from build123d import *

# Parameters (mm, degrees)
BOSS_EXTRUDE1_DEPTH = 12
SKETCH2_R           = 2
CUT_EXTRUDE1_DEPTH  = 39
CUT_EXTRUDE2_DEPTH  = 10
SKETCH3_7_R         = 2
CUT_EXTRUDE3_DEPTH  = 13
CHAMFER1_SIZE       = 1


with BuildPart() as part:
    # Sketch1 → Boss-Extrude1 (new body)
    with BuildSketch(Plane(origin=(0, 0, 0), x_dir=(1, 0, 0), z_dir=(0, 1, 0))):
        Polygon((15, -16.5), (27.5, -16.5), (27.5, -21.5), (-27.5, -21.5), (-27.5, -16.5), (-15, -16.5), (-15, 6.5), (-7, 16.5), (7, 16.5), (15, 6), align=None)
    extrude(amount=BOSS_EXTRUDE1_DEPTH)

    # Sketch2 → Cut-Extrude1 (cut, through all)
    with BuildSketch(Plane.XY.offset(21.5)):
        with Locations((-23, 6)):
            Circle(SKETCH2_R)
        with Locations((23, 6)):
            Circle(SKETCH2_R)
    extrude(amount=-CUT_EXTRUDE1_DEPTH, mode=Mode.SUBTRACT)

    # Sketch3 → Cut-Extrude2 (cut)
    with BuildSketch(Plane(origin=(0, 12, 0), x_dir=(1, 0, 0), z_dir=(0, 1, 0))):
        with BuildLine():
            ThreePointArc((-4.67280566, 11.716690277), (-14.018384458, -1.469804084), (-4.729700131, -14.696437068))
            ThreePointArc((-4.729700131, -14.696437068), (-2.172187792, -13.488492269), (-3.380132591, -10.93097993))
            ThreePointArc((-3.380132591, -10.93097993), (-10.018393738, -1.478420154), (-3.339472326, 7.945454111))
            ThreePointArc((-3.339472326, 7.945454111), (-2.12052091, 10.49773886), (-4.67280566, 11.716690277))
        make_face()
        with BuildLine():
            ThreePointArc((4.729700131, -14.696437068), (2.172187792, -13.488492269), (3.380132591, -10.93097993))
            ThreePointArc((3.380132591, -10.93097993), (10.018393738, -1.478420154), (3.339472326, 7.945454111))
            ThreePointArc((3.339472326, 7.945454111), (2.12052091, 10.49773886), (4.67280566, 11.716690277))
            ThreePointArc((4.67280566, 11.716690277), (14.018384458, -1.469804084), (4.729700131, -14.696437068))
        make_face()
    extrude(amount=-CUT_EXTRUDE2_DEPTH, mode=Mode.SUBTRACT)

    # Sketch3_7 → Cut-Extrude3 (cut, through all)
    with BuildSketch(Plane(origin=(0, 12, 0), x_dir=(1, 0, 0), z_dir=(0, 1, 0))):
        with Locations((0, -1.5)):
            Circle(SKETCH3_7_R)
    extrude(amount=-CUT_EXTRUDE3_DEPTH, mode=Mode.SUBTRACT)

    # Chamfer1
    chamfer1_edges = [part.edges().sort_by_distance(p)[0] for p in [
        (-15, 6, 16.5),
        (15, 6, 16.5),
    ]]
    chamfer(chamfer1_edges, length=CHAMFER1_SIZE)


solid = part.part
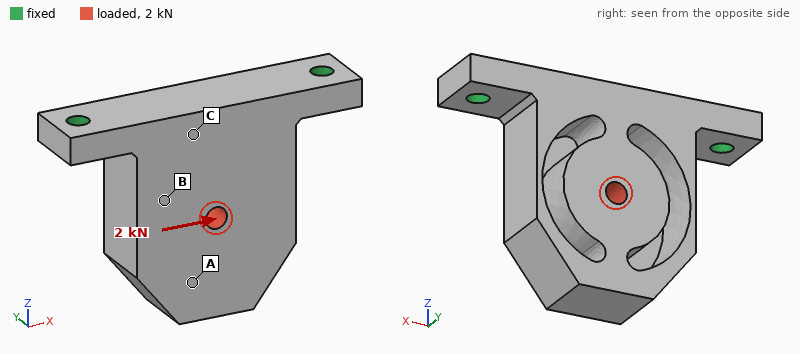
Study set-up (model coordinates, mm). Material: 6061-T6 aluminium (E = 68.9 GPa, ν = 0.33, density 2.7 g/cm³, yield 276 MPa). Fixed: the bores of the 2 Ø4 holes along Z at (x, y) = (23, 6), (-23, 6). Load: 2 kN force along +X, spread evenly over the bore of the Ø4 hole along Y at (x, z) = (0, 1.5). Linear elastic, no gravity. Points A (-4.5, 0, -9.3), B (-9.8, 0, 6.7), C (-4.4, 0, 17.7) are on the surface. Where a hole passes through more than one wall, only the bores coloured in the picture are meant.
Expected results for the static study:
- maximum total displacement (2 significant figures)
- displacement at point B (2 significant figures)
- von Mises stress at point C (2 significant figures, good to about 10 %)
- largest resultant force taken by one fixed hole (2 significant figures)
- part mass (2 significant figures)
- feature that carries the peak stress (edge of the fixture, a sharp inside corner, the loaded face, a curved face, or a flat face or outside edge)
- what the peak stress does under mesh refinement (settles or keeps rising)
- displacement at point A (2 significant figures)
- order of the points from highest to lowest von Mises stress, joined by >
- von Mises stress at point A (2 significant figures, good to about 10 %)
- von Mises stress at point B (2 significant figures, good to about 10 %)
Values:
69 µm
25 µm
23 MPa
1.4 kN
31 g
edge of the fixture
keeps rising
43 µm
B > C > A
9.9 MPa
34 MPa
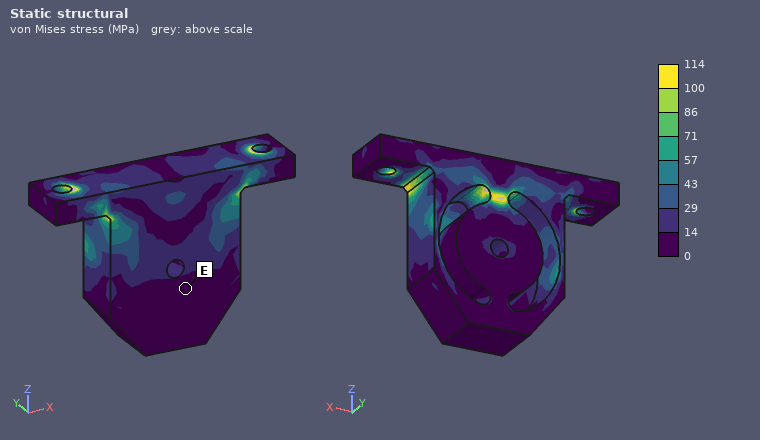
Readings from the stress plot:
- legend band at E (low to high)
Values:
0 to 14 MPa
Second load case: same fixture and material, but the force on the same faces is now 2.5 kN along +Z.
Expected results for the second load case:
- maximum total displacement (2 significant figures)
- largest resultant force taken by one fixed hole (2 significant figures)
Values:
47 µm
1.4 kN
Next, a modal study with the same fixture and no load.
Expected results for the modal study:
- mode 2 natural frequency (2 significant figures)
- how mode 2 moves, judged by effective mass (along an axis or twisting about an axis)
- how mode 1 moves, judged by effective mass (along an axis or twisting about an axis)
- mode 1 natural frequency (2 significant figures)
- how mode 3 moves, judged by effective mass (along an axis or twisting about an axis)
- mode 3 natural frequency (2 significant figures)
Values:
6800 Hz
along X
along Y
2500 Hz
along Z
8900 Hz
